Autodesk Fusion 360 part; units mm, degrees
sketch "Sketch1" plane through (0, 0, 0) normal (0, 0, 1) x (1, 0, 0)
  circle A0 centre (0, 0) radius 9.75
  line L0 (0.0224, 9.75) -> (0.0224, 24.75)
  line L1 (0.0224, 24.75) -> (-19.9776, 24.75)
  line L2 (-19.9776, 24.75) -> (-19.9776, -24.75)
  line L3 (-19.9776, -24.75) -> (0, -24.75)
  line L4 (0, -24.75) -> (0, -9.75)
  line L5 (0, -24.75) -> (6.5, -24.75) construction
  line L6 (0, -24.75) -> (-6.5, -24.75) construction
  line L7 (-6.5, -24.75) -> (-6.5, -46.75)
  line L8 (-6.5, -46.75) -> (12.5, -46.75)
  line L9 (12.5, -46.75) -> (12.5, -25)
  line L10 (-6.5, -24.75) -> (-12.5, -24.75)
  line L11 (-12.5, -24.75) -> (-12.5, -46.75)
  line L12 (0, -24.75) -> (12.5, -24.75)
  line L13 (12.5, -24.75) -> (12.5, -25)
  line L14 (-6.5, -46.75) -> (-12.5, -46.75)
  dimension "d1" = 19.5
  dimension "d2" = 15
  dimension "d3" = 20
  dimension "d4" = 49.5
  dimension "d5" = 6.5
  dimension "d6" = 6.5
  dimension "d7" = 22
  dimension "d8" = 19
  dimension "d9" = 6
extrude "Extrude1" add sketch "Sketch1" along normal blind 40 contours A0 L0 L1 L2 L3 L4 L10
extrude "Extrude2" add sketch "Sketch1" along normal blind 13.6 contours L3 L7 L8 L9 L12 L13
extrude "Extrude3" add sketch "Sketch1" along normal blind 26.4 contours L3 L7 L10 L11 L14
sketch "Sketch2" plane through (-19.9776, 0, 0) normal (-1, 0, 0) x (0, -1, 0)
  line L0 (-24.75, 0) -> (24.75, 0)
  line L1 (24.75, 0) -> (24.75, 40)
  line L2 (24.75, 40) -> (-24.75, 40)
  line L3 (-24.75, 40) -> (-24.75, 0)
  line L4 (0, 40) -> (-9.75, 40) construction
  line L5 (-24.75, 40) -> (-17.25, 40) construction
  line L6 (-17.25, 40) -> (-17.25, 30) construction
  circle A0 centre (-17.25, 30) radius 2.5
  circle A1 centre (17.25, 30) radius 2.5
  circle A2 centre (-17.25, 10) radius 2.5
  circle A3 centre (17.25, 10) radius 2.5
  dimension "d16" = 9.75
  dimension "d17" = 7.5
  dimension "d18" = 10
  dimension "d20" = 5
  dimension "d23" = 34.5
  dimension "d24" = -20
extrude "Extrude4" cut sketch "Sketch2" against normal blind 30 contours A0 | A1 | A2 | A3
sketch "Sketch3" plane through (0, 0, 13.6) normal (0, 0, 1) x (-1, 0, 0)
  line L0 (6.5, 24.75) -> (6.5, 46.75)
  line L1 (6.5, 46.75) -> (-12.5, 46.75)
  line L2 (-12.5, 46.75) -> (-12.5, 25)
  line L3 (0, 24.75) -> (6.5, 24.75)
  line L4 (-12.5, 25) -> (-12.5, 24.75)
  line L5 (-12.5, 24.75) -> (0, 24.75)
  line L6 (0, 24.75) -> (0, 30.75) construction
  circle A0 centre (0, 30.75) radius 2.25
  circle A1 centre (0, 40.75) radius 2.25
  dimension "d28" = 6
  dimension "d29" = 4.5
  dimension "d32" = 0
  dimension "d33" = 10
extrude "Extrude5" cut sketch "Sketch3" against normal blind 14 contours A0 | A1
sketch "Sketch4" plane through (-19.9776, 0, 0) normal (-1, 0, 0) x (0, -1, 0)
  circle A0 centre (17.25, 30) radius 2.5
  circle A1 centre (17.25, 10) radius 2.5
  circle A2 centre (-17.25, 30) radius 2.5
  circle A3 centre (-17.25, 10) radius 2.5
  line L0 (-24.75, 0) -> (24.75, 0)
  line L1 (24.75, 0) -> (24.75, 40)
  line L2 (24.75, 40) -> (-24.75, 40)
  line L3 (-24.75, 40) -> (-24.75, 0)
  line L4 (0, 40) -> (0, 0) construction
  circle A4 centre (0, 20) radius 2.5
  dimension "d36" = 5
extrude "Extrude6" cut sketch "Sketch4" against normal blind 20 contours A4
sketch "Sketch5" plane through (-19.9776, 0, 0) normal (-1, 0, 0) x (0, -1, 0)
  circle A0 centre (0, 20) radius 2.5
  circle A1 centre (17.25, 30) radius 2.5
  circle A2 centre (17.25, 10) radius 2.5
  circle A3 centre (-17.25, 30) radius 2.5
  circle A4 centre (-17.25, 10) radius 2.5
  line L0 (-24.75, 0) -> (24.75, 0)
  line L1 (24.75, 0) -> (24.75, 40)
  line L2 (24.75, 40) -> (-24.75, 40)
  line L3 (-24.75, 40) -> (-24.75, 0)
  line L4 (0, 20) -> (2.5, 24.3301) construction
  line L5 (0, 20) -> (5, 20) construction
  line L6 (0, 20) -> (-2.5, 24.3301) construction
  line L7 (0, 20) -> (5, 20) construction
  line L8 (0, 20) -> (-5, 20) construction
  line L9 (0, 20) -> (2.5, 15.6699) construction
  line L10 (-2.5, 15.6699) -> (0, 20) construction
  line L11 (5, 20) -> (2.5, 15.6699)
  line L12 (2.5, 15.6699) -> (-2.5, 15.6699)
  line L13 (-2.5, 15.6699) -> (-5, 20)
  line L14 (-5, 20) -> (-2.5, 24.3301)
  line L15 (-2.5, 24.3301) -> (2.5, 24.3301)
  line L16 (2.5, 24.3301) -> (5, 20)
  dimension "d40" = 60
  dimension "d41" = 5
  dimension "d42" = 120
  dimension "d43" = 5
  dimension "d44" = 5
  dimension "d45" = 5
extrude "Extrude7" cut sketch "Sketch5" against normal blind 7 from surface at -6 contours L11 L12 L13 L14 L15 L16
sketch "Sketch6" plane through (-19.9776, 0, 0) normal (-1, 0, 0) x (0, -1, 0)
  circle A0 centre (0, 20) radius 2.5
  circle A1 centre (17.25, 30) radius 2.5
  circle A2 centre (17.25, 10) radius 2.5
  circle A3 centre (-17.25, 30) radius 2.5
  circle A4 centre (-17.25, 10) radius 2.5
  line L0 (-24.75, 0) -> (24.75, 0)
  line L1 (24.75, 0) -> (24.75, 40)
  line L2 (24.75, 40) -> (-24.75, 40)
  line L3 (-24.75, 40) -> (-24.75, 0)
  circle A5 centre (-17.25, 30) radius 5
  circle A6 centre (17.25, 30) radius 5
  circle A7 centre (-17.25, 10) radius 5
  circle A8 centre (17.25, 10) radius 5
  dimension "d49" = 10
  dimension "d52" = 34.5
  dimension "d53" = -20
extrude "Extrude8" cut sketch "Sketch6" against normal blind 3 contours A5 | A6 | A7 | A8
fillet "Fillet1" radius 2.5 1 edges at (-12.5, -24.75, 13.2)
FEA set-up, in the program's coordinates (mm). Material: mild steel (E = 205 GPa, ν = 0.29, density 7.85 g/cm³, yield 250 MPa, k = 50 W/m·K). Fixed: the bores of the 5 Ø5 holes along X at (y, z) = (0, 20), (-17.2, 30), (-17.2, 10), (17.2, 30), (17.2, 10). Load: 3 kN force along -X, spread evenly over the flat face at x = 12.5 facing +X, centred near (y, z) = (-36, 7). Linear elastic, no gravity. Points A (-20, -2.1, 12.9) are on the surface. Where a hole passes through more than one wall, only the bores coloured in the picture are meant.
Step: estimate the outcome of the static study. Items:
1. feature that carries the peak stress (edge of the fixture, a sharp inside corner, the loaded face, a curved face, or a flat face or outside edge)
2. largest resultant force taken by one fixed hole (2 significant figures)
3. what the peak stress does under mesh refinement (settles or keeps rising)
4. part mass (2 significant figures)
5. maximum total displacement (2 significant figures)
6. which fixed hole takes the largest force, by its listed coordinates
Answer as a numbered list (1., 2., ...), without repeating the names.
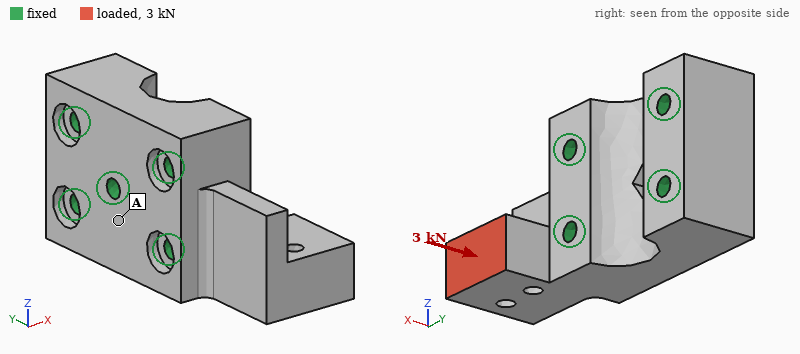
1. edge of the fixture
2. 3.1 kN
3. keeps rising
4. 310 g
5. 23 µm
6. (-17.2, 10)
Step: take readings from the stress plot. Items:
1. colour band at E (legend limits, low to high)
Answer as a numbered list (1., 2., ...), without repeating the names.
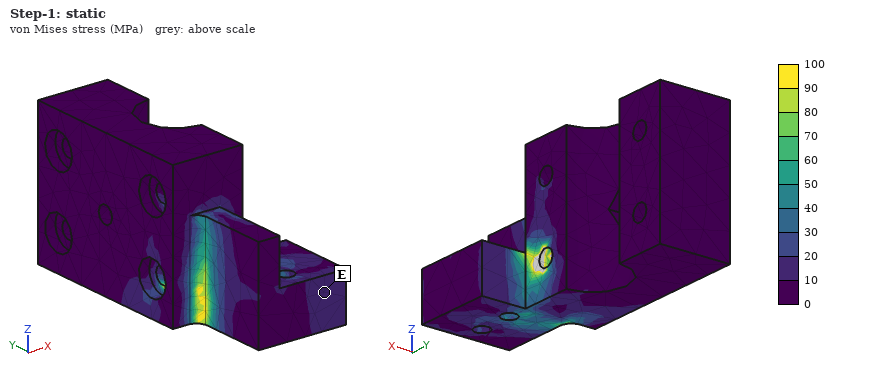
1. 10 to 20 MPa
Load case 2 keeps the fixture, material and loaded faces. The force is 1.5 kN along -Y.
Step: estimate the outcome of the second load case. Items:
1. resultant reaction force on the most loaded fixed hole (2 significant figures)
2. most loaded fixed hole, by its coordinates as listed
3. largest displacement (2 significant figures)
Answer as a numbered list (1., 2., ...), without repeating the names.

1. 1.8 kN
2. (-17.2, 10)
3. 19 µm
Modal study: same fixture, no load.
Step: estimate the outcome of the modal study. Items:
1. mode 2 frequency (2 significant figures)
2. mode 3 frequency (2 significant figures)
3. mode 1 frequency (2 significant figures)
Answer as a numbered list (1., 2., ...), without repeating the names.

1. 11 kHz
2. 18 kHz
3. 8400 Hz
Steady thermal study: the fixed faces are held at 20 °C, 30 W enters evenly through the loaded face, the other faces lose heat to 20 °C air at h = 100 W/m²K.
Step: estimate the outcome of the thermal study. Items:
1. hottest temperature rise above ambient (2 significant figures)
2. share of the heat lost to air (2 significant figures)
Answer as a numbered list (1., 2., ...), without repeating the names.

1. 59 K
2. 29 %
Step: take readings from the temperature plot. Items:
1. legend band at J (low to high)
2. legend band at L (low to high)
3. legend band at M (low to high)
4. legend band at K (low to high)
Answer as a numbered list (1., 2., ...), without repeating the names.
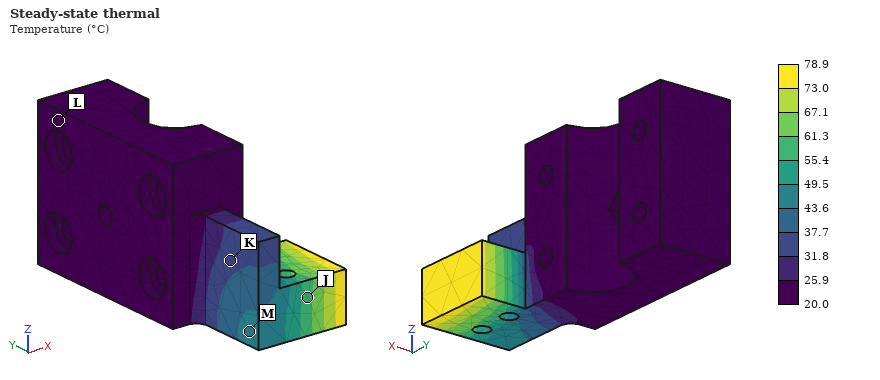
1. 55.4 to 61.3 °C
2. 20.0 to 25.9 °C
3. 43.6 to 49.5 °C
4. 31.8 to 37.7 °C
